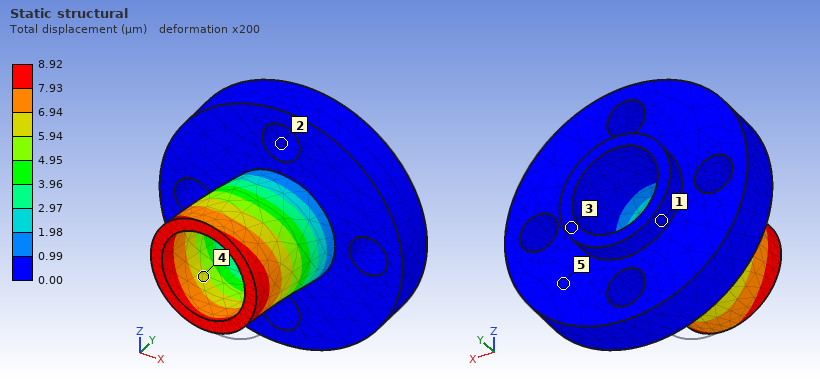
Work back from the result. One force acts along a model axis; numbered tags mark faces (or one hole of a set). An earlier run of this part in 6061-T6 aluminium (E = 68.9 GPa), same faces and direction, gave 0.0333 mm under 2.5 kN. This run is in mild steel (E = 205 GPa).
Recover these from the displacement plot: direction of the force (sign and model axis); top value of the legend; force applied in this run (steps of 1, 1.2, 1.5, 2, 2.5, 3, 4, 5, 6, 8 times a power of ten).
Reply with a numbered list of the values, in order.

1. -X
2. 8.92 µm
3. 2 kN
